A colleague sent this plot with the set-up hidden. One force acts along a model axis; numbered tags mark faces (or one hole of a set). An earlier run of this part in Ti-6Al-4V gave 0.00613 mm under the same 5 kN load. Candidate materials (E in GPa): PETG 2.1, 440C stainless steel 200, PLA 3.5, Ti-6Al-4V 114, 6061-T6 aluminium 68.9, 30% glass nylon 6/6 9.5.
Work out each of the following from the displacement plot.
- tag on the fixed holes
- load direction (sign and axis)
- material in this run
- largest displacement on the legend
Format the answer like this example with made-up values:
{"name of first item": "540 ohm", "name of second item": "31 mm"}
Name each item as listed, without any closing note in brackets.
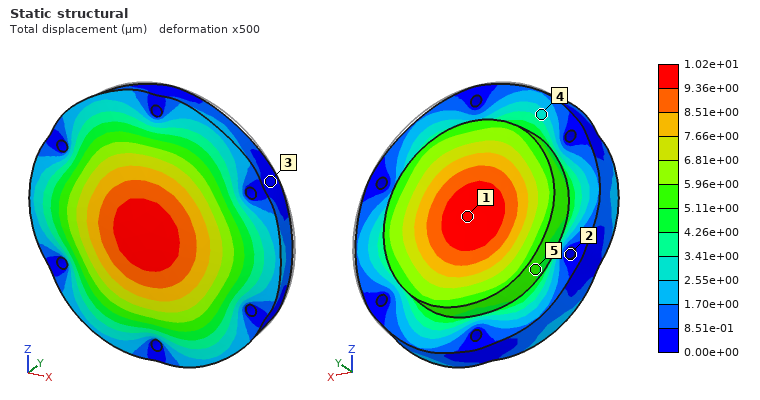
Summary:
{"tag on the fixed holes": "2", "load direction": "-Y", "material in this run": "6061-T6 aluminium", "largest displacement on the legend": "1.02e+01 µm"}
